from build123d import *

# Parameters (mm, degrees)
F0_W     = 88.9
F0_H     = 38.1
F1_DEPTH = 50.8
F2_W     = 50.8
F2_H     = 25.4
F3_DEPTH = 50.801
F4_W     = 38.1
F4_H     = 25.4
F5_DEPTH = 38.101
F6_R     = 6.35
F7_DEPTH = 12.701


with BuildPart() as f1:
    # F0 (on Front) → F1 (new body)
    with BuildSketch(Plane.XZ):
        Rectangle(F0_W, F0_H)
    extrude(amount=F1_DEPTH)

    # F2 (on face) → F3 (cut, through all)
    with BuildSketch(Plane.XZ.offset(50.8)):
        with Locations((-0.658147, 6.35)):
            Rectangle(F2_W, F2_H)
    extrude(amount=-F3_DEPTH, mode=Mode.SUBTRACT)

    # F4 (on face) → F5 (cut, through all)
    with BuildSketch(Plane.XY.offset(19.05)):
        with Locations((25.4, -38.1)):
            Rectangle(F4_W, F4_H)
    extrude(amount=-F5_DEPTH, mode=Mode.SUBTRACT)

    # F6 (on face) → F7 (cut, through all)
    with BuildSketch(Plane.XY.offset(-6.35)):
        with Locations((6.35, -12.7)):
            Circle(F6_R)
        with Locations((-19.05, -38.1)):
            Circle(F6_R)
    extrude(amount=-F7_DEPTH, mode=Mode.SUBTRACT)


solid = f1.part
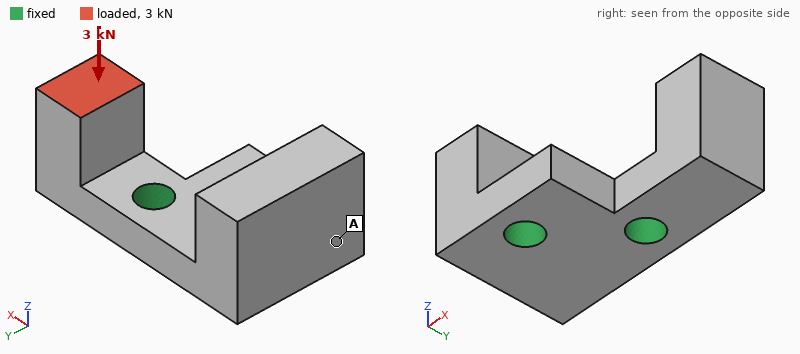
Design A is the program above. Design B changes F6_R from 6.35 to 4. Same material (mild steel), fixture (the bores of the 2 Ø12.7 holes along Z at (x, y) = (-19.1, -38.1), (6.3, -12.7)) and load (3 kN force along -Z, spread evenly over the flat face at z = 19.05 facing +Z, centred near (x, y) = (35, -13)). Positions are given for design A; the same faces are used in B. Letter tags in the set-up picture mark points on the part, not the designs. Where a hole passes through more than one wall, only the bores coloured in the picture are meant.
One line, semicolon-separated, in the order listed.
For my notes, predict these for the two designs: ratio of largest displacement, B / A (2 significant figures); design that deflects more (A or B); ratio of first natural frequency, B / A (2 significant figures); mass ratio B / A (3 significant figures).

1.3; B; 0.89; 1.02
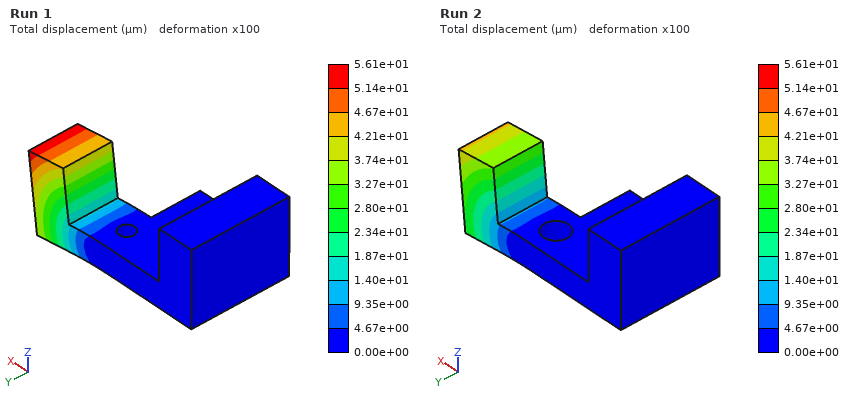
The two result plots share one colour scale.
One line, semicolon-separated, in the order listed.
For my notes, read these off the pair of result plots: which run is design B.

Run 1
